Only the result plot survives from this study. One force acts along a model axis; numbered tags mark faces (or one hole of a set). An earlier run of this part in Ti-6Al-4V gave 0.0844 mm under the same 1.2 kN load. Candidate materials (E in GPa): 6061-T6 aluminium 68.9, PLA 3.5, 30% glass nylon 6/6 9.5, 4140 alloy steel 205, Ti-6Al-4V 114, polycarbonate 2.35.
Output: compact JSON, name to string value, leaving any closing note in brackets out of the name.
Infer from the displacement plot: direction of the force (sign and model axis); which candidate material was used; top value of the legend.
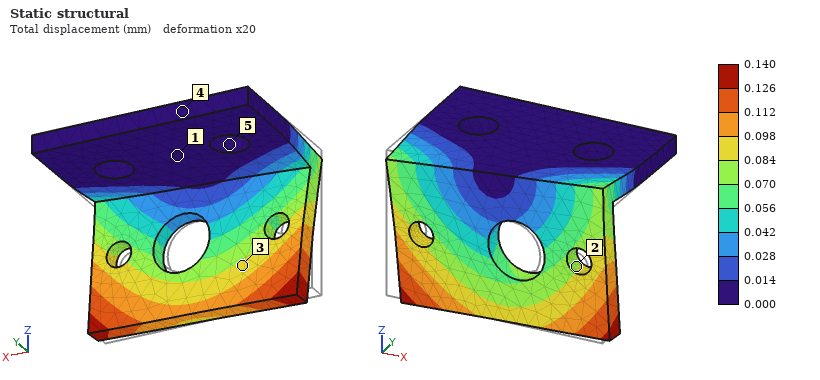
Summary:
{"direction of the force": "+X", "which candidate material was used": "6061-T6 aluminium", "top value of the legend": "0.140 mm"}
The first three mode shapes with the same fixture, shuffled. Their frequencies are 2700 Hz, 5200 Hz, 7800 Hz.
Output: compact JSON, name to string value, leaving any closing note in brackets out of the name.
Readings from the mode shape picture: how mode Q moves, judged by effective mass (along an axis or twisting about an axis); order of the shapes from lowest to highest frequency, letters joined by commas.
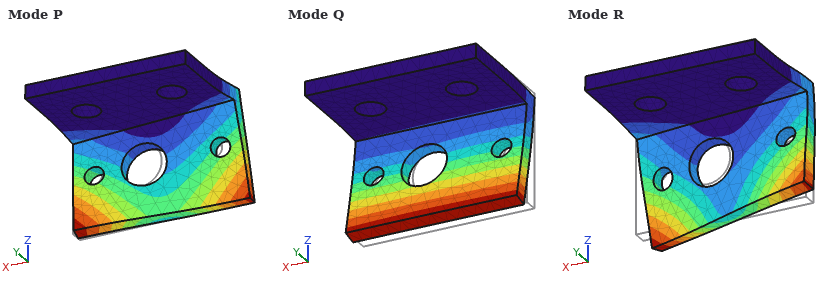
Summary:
{"how mode Q moves, judged by effective mass": "along Y", "order of the shapes from lowest to highest frequency, letters joined by commas": "Q, P, R"}
